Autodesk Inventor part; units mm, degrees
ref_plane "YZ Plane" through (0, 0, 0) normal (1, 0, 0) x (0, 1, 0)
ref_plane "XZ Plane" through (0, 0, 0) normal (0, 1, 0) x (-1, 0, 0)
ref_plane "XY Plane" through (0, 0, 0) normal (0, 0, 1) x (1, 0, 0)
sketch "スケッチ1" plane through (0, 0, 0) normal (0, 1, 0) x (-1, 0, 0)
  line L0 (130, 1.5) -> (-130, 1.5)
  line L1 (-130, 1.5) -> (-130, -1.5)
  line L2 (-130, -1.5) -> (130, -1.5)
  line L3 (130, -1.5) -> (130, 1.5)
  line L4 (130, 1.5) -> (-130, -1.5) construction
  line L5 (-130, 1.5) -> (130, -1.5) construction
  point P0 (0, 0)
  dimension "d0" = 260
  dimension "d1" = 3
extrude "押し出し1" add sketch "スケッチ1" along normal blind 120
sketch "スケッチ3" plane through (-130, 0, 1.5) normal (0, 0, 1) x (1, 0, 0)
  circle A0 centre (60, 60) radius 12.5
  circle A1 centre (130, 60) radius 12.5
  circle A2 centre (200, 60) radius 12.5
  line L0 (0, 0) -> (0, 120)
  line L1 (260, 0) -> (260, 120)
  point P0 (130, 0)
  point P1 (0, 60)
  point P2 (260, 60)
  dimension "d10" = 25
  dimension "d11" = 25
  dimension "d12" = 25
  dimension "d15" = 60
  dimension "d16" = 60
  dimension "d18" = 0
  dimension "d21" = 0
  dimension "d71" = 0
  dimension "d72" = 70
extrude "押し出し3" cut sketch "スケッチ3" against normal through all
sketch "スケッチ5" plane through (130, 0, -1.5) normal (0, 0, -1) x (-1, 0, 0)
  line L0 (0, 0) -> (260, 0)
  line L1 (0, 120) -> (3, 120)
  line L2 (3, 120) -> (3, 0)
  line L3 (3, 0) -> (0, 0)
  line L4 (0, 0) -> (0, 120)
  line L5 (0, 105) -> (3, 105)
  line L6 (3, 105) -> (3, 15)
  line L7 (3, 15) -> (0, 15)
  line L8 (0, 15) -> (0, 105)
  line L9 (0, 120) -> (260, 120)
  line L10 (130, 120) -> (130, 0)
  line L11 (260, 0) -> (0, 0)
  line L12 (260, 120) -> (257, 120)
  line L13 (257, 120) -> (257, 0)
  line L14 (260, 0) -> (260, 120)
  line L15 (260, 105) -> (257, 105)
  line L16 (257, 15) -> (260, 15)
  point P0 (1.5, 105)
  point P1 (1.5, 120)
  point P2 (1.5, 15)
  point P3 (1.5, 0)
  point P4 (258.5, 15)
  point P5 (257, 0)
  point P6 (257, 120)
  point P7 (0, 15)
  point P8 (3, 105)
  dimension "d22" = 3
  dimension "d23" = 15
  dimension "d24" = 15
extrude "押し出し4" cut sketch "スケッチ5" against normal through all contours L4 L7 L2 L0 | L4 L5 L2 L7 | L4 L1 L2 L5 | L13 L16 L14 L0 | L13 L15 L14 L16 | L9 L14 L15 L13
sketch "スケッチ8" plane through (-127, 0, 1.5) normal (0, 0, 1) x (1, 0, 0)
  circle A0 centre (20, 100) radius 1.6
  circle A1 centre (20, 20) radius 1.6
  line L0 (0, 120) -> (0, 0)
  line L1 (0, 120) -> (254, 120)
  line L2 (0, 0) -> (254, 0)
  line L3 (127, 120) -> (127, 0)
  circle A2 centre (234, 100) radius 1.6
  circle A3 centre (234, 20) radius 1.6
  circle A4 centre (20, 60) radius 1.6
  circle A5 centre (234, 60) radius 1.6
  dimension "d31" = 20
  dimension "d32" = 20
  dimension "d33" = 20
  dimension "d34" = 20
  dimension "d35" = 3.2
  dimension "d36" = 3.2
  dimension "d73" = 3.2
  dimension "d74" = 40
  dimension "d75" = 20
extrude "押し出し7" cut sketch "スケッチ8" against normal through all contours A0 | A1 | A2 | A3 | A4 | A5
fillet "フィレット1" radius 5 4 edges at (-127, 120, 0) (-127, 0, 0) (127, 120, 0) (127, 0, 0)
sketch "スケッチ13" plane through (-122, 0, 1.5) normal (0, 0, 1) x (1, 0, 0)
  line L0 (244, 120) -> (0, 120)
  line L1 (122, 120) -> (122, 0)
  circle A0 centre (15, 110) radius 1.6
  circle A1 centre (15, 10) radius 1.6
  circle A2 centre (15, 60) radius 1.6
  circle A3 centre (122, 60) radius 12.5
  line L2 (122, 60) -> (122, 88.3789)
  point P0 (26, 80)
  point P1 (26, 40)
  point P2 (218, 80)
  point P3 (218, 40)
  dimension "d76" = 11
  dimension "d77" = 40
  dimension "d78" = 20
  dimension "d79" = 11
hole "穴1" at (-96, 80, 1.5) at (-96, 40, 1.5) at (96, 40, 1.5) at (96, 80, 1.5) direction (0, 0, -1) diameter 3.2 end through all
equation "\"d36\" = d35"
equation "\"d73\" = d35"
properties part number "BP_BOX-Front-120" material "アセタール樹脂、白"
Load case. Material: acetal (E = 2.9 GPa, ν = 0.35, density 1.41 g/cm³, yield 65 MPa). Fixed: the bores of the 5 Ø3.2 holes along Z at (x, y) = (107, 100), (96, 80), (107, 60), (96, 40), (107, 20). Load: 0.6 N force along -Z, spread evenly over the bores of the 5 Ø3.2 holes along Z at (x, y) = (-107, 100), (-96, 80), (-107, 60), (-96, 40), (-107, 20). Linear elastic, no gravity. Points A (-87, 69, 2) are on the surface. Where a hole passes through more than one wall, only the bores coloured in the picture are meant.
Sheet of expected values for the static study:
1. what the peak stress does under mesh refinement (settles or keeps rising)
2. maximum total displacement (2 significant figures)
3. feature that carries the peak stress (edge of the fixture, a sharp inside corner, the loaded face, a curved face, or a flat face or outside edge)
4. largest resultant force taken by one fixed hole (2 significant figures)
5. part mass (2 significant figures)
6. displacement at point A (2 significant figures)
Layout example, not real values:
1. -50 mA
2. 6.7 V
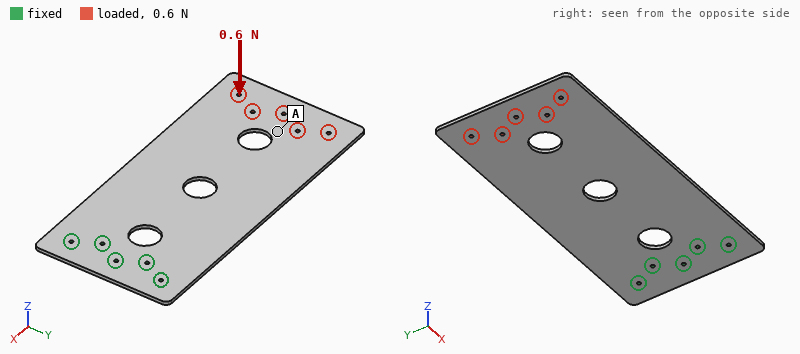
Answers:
1. keeps rising
2. 2.7 mm
3. edge of the fixture
4. 2.3 N
5. 120 g
6. 2.0 mm
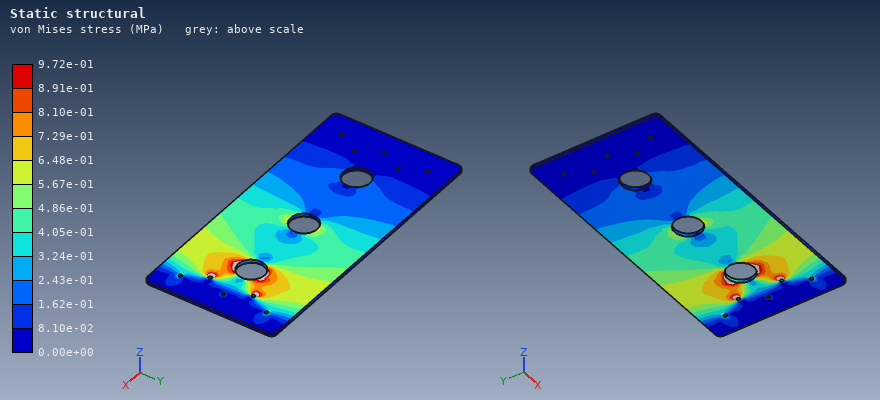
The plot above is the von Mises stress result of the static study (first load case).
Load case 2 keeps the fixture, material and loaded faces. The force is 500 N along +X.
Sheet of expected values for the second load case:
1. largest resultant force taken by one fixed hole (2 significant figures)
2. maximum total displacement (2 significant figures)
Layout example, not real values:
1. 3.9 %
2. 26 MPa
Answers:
1. 130 N
2. 0.14 mm
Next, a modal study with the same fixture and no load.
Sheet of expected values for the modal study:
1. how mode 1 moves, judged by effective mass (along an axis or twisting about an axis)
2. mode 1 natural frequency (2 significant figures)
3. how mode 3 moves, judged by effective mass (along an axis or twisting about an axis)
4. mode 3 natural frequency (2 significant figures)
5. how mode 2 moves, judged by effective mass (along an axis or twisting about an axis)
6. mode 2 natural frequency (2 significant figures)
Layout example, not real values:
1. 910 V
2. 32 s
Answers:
1. along Z
2. 13 Hz
3. along Z
4. 83 Hz
5. twisting about X
6. 52 Hz
